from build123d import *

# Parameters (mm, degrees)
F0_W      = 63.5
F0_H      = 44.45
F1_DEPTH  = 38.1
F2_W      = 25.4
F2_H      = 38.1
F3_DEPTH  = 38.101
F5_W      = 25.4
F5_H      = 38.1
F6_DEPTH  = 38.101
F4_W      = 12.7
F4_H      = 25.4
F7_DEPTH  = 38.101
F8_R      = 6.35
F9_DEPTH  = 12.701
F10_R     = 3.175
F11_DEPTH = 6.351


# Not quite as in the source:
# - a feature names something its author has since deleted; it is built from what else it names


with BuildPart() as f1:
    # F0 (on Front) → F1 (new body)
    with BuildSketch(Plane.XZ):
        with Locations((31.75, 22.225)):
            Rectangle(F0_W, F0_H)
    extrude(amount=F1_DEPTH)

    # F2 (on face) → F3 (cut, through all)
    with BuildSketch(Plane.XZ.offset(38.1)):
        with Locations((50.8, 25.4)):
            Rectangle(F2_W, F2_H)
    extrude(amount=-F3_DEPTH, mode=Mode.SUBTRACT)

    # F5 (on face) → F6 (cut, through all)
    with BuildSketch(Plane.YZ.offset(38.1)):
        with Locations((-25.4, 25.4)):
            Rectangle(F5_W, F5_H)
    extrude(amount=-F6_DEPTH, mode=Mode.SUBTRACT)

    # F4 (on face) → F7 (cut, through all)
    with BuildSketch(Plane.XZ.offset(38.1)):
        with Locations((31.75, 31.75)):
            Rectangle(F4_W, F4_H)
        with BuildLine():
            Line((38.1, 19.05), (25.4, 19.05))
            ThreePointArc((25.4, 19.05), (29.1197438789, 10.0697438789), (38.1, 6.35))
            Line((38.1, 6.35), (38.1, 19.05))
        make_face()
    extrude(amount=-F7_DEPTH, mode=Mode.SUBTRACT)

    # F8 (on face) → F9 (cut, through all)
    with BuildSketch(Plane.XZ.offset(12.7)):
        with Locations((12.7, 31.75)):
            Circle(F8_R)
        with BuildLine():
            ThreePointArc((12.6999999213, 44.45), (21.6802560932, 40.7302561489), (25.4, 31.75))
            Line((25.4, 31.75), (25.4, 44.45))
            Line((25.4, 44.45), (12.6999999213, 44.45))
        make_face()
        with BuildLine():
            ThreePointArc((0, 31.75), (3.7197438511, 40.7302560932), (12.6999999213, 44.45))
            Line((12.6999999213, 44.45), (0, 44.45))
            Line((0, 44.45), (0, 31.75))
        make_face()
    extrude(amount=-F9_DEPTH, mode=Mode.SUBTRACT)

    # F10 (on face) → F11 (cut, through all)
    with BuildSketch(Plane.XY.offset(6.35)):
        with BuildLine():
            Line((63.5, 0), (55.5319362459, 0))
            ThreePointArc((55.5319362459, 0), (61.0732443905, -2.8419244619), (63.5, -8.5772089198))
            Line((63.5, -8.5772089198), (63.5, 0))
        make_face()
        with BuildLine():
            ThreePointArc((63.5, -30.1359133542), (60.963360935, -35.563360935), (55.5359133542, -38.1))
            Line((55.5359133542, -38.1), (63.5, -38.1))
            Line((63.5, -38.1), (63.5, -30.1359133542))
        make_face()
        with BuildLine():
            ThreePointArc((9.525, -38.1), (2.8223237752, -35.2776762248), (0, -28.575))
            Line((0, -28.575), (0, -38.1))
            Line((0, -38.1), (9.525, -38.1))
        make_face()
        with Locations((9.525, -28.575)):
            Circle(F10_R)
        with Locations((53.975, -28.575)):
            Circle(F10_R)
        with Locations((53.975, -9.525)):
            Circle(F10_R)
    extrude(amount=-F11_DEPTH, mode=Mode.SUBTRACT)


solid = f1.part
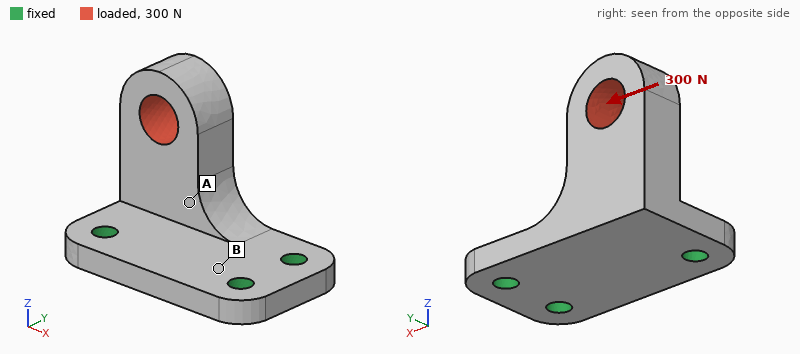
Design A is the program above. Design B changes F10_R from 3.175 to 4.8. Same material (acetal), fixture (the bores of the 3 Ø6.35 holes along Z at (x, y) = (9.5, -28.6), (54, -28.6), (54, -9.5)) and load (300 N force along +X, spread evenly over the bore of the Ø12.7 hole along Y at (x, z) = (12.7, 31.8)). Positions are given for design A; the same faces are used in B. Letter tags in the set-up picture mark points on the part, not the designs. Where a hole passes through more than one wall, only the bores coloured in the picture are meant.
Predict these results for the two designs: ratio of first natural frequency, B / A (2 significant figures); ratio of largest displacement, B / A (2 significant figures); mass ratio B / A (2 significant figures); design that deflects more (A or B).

1.1
0.85
0.97
A
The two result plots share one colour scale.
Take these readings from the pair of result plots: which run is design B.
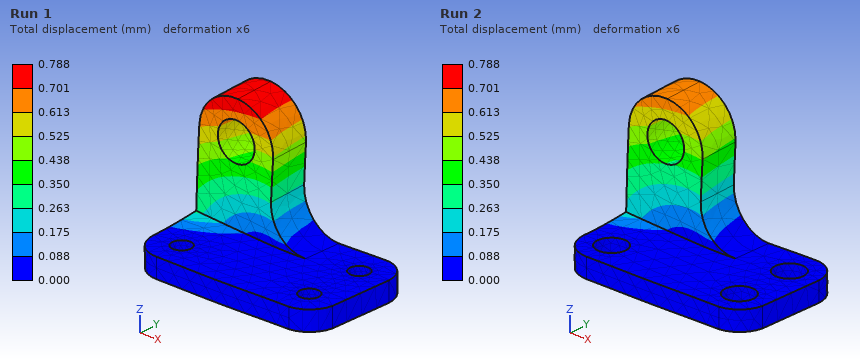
Run 2
